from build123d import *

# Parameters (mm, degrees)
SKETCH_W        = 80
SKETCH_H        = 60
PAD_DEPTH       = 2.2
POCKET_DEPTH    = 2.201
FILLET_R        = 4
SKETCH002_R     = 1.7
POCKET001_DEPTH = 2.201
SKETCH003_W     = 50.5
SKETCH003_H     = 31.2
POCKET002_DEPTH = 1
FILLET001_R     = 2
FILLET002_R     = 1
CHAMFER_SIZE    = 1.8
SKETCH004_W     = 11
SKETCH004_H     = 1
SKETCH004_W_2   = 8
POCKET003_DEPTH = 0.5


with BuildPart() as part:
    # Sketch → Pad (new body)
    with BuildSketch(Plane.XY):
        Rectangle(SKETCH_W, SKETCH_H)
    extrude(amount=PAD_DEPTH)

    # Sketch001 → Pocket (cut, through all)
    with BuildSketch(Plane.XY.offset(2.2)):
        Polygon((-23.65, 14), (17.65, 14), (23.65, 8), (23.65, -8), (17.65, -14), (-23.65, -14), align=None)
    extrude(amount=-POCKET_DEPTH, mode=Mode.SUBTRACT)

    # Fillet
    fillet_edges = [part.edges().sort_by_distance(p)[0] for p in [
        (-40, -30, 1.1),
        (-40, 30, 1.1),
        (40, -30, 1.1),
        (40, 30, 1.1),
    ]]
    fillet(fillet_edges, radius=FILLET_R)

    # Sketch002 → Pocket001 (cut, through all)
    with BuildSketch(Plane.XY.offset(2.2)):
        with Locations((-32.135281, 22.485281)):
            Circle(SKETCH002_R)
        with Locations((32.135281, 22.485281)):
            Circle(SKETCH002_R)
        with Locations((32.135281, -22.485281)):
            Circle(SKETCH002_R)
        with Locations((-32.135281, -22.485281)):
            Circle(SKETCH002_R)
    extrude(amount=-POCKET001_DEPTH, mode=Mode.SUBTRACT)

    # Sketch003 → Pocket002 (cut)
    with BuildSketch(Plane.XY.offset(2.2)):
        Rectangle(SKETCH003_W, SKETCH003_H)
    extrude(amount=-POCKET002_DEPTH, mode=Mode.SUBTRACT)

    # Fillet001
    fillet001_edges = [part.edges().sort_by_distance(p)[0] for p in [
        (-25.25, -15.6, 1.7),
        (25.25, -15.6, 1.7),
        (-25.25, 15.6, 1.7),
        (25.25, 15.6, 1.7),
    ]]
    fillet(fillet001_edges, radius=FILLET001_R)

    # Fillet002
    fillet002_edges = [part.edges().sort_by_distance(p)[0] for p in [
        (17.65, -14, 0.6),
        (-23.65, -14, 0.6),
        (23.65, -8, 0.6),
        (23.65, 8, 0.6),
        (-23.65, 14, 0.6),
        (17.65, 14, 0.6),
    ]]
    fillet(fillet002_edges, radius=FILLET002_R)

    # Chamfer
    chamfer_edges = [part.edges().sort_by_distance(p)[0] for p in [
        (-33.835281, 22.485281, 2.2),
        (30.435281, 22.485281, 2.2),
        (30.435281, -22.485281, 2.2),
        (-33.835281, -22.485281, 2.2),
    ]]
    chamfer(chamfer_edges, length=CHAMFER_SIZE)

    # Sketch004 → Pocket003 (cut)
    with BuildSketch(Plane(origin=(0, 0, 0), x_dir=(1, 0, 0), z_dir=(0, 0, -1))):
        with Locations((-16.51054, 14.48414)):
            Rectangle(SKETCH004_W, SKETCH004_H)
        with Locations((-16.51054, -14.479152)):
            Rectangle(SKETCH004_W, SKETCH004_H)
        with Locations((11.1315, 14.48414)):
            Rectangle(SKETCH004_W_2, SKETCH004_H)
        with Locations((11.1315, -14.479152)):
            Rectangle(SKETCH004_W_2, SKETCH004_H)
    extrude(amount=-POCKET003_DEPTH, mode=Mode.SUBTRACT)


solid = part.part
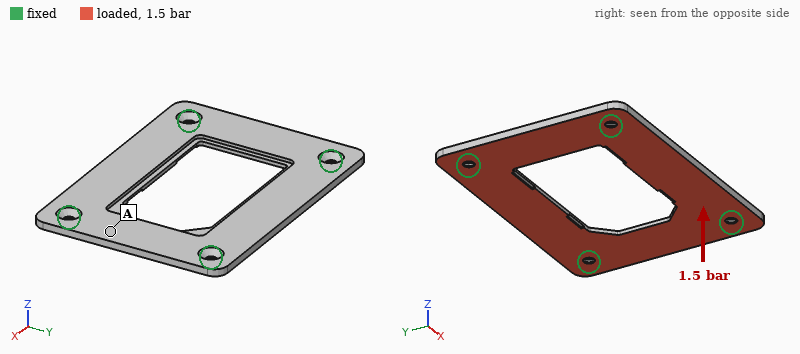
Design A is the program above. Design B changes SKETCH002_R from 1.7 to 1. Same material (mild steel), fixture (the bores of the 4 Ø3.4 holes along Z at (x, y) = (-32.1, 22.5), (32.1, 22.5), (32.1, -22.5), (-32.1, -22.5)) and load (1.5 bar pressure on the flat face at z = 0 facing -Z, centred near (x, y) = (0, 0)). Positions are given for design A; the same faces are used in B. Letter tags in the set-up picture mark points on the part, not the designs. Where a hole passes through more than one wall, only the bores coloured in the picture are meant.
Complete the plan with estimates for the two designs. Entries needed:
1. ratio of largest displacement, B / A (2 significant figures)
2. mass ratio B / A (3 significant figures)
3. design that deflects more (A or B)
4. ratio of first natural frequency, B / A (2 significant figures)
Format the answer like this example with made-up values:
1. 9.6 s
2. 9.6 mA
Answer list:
1. 1.3
2. 1.01
3. B
4. 0.87
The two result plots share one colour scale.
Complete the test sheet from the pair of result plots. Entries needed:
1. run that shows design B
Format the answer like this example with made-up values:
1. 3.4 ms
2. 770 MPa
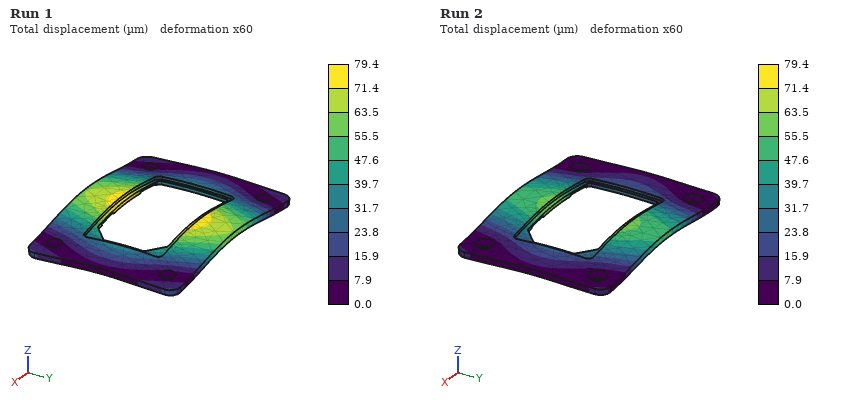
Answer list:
1. Run 1
